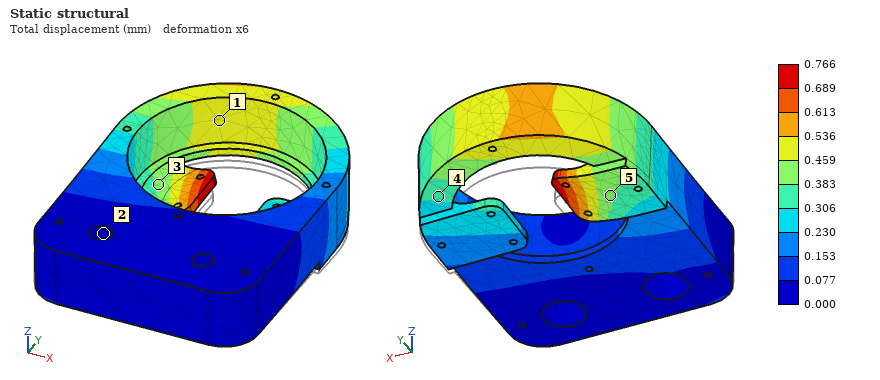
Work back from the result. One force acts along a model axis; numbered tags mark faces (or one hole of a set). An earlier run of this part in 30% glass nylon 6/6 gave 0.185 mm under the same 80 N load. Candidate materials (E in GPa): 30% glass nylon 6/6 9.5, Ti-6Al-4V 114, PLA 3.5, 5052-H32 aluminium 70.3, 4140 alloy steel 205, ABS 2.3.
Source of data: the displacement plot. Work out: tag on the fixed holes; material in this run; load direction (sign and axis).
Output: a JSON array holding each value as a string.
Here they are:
["2", "ABS", "+Z"]
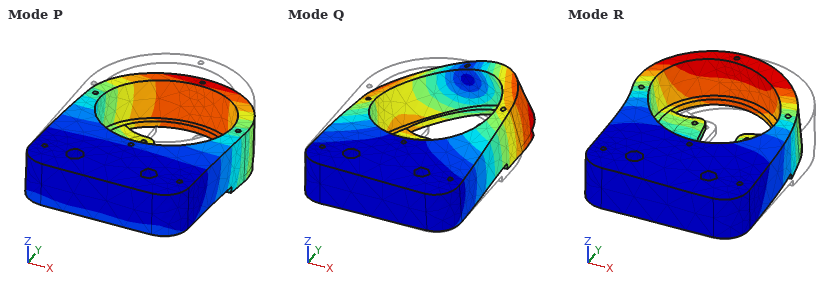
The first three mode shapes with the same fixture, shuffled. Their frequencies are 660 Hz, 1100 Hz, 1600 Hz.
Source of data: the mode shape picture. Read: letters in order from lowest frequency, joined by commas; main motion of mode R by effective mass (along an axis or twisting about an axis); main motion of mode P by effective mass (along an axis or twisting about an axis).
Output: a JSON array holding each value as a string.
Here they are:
["P, R, Q", "along X", "along Z"]
